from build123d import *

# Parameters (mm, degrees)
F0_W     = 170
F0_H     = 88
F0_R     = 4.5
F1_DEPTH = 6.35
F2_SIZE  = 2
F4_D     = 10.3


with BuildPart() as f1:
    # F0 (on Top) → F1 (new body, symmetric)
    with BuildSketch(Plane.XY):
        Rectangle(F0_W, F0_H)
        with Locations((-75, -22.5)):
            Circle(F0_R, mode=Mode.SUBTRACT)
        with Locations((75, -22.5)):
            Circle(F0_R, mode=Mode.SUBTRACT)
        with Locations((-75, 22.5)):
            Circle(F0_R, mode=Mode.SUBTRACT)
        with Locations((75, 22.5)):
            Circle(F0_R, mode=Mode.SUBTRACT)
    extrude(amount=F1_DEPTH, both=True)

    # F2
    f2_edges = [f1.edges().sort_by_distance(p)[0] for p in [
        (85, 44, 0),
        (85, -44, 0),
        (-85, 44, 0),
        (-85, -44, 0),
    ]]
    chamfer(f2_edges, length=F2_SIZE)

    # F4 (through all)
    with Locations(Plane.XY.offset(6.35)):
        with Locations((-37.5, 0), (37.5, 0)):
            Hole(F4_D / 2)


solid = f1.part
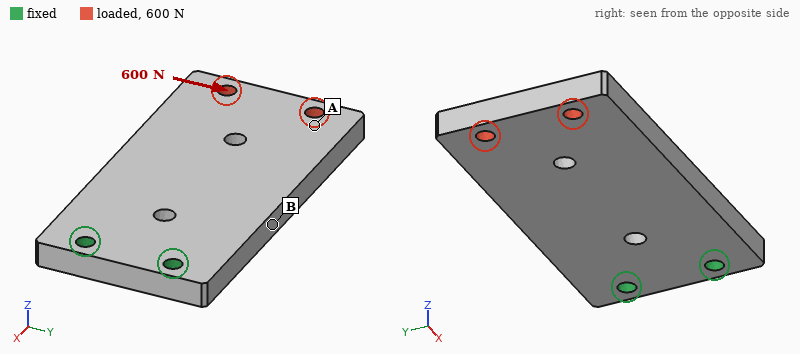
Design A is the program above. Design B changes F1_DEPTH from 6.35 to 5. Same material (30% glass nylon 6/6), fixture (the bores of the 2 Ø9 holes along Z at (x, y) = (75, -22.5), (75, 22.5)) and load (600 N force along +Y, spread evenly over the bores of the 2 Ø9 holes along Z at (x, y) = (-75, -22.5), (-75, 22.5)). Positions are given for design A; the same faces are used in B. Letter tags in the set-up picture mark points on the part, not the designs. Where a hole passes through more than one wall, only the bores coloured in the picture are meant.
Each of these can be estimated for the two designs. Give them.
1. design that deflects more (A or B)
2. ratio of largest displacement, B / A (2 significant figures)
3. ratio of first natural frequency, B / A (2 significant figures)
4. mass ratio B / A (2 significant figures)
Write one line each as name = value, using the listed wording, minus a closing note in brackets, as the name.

design that deflects more = B
ratio of largest displacement, B / A = 1.3
ratio of first natural frequency, B / A = 0.80
mass ratio B / A = 0.79
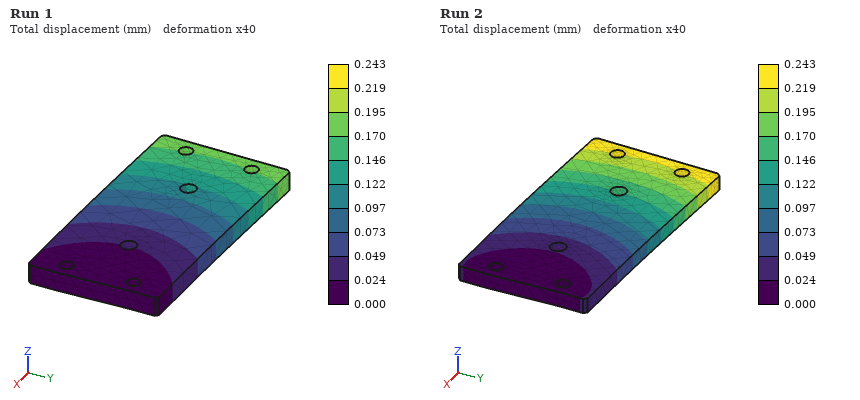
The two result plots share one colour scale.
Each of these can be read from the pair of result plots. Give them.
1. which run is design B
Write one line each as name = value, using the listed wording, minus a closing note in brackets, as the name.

which run is design B = Run 2
